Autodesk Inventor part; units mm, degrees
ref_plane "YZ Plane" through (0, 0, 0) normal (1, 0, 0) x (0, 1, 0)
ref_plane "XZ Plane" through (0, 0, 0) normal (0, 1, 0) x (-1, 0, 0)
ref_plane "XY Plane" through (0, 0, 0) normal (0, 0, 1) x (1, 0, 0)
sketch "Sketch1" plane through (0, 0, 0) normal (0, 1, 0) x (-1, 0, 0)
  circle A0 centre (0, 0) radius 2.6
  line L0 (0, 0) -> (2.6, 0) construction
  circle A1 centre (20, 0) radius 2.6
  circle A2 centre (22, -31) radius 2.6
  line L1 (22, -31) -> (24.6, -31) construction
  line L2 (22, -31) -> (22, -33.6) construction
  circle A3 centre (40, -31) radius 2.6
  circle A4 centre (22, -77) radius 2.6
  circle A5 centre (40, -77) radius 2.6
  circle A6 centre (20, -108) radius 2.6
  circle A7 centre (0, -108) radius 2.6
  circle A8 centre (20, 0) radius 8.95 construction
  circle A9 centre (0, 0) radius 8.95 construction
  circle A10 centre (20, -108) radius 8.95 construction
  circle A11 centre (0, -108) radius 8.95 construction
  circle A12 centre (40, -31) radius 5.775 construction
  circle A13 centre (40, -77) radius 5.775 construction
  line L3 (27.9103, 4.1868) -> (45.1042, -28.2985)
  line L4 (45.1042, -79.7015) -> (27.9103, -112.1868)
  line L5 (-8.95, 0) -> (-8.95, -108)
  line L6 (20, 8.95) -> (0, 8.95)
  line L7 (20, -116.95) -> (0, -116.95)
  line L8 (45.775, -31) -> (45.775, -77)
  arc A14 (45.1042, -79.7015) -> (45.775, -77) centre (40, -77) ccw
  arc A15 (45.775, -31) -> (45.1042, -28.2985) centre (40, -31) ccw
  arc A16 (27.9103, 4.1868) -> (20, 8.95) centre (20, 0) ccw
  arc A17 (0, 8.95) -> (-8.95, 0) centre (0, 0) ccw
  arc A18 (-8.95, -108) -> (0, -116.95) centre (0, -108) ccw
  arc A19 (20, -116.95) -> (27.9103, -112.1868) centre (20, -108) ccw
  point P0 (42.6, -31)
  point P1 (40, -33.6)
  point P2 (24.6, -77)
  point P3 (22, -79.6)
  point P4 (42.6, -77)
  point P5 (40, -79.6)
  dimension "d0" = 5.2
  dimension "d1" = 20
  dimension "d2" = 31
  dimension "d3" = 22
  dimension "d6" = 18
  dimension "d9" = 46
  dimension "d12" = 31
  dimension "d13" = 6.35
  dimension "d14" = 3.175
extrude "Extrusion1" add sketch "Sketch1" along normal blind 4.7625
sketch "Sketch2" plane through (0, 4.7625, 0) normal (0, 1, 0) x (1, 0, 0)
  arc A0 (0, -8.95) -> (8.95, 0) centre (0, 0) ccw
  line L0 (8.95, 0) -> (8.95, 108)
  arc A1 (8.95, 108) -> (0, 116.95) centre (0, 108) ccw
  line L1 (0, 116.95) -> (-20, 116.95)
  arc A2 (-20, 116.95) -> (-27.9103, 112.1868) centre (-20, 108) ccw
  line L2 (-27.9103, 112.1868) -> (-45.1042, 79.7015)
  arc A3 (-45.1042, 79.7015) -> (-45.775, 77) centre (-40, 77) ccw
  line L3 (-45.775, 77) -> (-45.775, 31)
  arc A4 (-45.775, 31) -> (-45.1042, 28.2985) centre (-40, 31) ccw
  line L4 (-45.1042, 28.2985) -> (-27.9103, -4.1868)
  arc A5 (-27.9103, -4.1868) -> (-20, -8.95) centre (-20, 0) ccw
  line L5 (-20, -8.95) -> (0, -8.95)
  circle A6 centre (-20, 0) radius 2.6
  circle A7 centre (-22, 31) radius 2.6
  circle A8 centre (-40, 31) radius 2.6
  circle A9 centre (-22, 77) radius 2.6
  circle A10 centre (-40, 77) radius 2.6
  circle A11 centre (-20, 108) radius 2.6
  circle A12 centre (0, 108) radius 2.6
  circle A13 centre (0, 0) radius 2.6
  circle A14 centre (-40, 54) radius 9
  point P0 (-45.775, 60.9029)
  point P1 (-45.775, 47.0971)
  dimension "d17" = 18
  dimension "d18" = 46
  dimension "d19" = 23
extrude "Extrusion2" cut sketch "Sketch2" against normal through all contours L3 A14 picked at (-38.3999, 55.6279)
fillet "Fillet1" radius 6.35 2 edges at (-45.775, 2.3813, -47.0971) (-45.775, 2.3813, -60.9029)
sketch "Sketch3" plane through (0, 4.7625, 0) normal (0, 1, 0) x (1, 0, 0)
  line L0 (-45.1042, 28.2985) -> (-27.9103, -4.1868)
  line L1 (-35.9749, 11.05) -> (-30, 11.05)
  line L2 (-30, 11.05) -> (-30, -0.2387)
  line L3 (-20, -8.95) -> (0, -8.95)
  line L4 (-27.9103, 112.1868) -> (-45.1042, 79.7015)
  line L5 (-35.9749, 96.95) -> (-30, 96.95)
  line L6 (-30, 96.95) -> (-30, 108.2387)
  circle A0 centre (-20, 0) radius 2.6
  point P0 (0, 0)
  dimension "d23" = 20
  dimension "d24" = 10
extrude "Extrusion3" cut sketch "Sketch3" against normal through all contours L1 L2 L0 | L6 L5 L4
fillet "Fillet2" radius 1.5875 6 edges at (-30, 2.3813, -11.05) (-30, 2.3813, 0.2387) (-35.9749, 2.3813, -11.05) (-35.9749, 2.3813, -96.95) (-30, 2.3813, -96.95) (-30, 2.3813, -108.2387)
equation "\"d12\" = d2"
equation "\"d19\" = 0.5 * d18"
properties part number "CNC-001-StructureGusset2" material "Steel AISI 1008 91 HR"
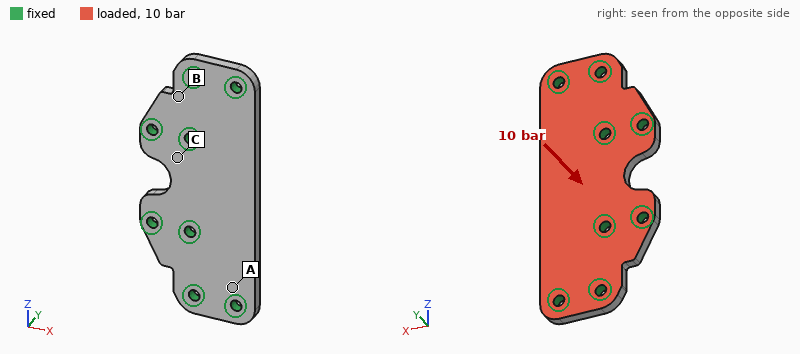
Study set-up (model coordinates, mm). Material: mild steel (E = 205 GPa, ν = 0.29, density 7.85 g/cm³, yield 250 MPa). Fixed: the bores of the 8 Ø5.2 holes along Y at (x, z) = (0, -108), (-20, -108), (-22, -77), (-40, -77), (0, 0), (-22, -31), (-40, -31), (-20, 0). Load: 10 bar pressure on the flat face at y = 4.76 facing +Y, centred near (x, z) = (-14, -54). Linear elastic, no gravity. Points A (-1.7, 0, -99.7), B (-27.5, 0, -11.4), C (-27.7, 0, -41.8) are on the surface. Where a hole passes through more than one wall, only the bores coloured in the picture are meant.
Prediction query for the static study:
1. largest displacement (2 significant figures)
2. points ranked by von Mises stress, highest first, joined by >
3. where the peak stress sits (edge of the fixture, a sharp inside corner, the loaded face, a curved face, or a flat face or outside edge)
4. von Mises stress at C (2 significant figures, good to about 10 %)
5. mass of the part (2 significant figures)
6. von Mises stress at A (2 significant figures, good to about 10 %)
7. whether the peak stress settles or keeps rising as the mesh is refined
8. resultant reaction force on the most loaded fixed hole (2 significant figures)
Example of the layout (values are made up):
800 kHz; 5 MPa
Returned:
55 µm; A > C > B; edge of the fixture; 26 MPa; 210 g; 39 MPa; keeps rising; 1.5 kN
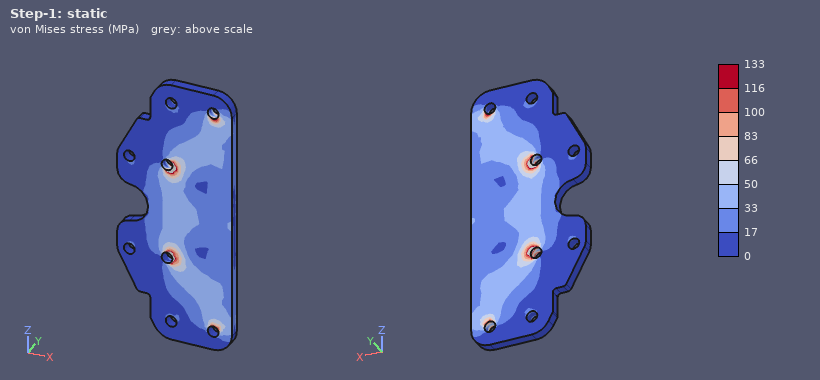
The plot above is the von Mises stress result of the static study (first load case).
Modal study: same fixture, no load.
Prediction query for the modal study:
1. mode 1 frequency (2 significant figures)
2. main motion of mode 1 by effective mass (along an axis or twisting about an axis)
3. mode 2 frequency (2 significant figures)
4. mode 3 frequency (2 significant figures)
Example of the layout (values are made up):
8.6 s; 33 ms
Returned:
4800 Hz; along Y; 8800 Hz; 12 kHz
